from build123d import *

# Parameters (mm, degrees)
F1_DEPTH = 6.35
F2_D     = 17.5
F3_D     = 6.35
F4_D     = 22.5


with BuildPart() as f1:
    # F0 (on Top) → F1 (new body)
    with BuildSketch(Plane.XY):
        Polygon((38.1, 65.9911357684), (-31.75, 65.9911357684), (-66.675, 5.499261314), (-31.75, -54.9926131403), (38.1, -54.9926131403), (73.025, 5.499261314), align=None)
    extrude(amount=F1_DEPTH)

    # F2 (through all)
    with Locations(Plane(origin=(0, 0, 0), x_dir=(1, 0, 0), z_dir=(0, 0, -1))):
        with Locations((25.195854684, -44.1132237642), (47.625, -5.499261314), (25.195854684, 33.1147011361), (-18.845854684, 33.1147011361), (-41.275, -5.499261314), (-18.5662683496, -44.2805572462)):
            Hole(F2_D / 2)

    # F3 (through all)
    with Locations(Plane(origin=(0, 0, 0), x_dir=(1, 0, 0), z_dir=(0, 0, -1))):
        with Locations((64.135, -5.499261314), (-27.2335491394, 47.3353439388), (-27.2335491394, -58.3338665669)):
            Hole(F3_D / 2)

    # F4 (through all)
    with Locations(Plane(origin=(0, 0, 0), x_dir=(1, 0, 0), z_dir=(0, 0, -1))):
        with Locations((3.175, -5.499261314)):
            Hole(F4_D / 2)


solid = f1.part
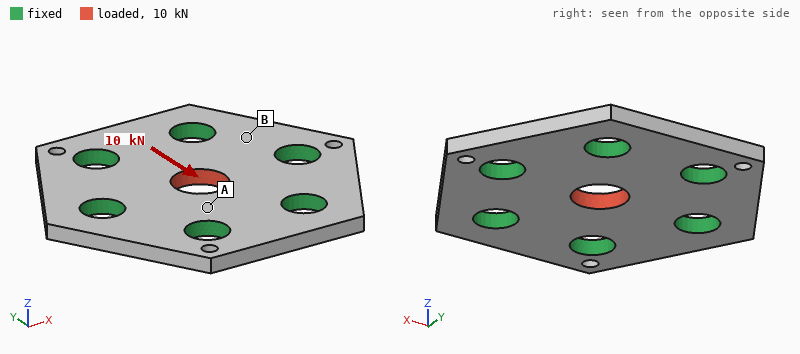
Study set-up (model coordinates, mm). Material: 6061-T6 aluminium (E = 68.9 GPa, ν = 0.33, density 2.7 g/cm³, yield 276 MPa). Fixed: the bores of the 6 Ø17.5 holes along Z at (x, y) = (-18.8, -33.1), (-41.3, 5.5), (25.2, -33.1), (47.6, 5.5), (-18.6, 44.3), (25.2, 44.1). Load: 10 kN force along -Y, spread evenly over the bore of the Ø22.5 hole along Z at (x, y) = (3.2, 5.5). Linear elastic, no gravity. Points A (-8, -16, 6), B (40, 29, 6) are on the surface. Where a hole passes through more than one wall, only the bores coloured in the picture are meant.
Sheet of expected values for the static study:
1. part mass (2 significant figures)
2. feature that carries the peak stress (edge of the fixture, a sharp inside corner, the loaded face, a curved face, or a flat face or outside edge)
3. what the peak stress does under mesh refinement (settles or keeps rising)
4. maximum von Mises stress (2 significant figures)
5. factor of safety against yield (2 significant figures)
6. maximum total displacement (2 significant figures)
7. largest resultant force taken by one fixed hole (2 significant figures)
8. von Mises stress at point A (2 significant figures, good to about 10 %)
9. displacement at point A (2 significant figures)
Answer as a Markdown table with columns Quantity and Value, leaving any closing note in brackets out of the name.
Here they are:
| Quantity | Value |
|---|---|
| part mass | 180 g |
| feature that carries the peak stress | the loaded face |
| what the peak stress does under mesh refinement | settles |
| maximum von Mises stress | 39 MPa |
| factor of safety against yield | 7.1 |
| maximum total displacement | 7.6 µm |
| largest resultant force taken by one fixed hole | 2.4 kN |
| von Mises stress at point A | 17 MPa |
| displacement at point A | 3.2 µm |
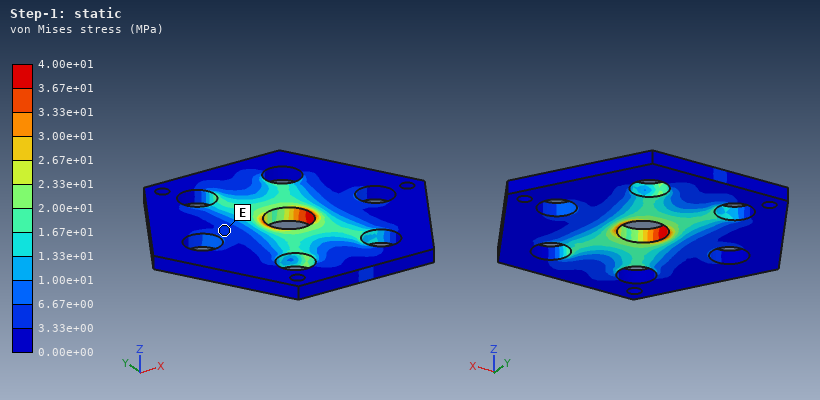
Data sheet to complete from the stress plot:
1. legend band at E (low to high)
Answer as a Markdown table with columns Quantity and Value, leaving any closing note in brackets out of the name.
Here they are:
| Quantity | Value |
|---|---|
| legend band at E | 3.33e+00 to 6.67e+00 MPa |
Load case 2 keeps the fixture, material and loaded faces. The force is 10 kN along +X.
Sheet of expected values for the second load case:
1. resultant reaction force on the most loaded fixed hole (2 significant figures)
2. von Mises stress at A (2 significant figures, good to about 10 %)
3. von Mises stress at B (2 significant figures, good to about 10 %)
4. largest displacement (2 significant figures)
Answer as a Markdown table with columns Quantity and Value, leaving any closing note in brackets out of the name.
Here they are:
| Quantity | Value |
|---|---|
| resultant reaction force on the most loaded fixed hole | 2.8 kN |
| von Mises stress at A | 11 MPa |
| von Mises stress at B | 3.7 MPa |
| largest displacement | 7.5 µm |
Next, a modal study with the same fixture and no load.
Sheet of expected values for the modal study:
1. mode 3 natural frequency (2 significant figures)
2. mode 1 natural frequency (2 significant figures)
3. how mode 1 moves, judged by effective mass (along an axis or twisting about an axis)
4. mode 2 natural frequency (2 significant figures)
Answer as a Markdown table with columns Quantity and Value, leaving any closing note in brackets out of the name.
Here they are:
| Quantity | Value |
|---|---|
| mode 3 natural frequency | 16 kHz |
| mode 1 natural frequency | 11 kHz |
| how mode 1 moves, judged by effective mass | along Z |
| mode 2 natural frequency | 16 kHz |
